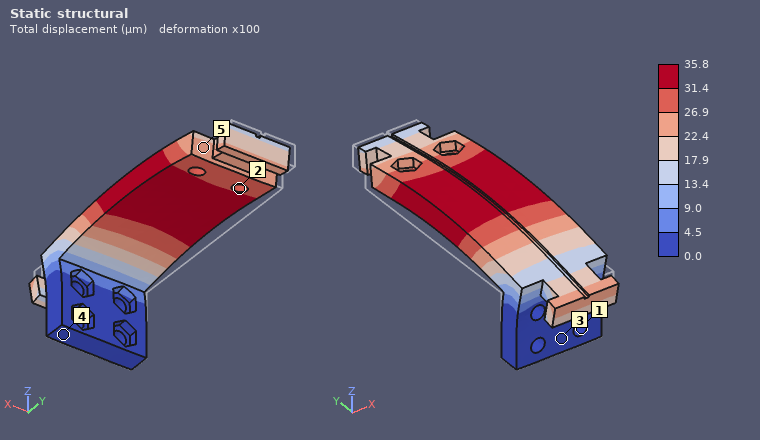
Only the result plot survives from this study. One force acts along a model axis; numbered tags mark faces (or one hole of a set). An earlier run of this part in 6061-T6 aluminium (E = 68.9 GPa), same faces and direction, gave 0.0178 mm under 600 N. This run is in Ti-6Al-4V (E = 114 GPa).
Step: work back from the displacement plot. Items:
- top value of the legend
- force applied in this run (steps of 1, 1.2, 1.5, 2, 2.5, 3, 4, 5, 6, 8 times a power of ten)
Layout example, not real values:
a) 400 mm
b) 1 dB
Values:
a) 35.8 µm
b) 2 kN
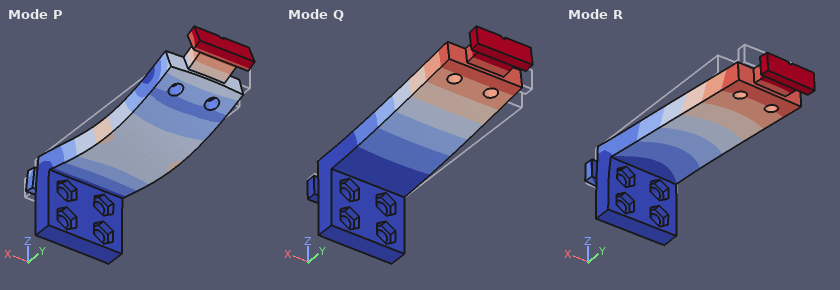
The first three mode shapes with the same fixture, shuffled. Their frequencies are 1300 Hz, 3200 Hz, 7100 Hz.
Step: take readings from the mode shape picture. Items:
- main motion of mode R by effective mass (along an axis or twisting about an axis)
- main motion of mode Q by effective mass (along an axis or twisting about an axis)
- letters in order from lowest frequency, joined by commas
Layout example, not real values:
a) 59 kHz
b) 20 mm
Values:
a) along X
b) along Z
c) Q, R, P
